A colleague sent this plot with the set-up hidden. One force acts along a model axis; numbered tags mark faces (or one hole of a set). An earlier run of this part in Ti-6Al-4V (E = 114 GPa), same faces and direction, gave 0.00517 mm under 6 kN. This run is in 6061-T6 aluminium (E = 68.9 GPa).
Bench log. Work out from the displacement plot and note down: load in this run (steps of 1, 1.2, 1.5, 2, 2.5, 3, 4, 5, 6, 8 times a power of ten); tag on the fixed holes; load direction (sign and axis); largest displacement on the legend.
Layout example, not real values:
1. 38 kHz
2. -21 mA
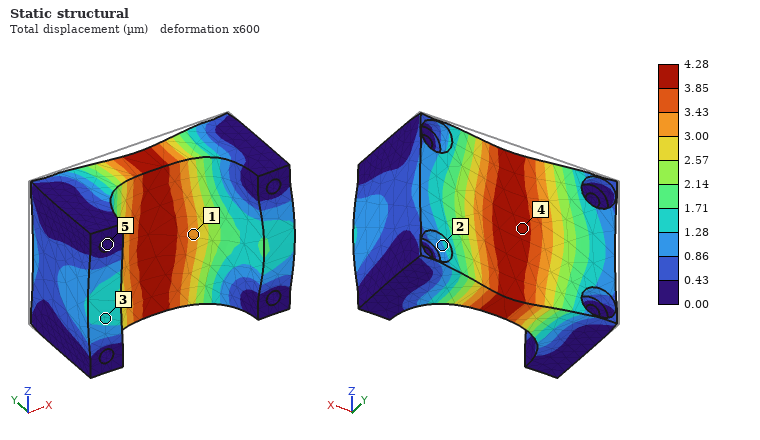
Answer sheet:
1. 3 kN
2. 5
3. -Y
4. 4.28 µm
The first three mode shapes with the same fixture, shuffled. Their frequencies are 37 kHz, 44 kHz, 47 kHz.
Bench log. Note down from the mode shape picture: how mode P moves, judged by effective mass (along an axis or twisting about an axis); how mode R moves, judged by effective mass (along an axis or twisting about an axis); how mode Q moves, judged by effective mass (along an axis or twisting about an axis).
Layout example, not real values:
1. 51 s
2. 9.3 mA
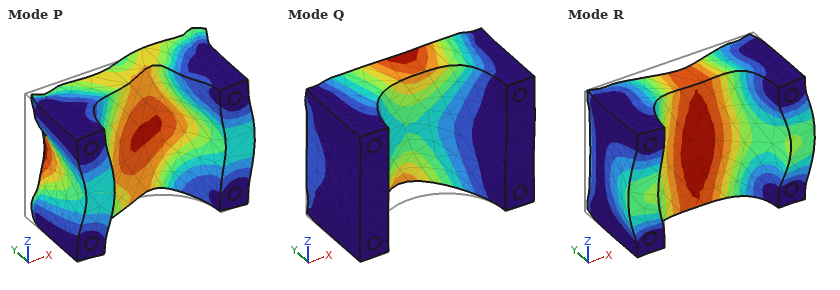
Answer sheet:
1. along X
2. along Y
3. along Z
